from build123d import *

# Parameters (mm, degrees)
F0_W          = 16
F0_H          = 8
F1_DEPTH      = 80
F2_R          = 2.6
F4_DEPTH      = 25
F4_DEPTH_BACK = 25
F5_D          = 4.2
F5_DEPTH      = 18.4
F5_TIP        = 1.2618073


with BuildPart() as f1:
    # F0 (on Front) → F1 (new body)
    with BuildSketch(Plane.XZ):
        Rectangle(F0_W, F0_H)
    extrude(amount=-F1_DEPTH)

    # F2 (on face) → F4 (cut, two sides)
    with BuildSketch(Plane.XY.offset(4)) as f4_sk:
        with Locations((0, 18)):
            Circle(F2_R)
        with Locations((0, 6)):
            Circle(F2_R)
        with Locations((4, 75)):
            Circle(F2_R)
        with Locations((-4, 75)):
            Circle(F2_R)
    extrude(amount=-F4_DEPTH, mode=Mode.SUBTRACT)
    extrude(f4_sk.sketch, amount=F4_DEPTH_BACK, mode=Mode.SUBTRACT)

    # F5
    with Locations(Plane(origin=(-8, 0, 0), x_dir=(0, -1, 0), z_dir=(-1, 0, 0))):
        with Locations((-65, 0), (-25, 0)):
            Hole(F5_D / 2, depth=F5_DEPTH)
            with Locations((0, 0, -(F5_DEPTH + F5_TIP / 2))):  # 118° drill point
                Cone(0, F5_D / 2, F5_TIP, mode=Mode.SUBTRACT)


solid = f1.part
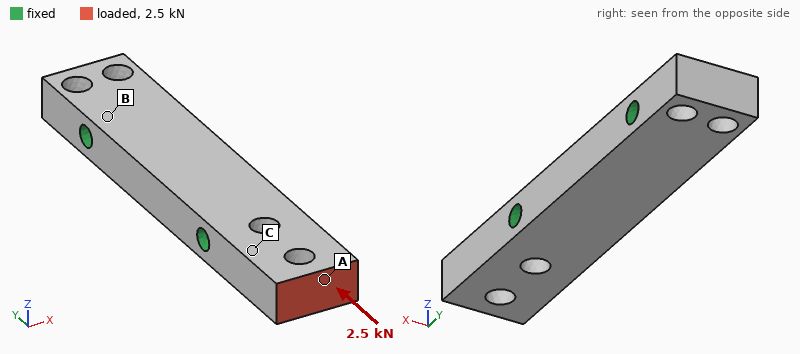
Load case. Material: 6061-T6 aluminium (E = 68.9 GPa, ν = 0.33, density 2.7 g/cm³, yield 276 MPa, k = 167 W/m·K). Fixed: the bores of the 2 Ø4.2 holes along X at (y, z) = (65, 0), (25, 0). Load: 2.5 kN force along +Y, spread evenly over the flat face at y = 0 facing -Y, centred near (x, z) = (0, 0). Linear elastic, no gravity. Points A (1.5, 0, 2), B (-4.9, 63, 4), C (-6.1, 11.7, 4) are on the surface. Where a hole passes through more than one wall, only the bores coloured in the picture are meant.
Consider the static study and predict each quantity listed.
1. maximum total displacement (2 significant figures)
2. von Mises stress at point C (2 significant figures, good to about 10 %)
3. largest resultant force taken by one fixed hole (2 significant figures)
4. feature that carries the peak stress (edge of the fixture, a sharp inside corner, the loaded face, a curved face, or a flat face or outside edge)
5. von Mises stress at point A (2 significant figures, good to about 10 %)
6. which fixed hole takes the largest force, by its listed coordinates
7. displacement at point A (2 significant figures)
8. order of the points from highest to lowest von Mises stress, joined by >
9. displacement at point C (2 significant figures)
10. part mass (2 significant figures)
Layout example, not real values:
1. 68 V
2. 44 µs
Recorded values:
1. 11 µm
2. 27 MPa
3. 2.5 kN
4. a curved face
5. 18 MPa
6. (25, 0)
7. 10 µm
8. C > A > B
9. 4.7 µm
10. 25 g
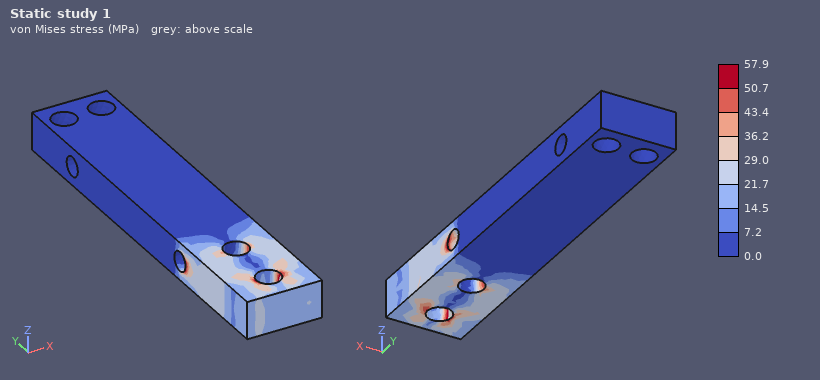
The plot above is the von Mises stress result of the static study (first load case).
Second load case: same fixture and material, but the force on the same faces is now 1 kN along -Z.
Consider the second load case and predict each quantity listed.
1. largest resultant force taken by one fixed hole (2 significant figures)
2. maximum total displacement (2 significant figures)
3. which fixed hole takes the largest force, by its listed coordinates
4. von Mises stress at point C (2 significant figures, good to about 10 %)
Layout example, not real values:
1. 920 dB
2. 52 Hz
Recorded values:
1. 1.1 kN
2. 0.16 mm
3. (25, 0)
4. 86 MPa
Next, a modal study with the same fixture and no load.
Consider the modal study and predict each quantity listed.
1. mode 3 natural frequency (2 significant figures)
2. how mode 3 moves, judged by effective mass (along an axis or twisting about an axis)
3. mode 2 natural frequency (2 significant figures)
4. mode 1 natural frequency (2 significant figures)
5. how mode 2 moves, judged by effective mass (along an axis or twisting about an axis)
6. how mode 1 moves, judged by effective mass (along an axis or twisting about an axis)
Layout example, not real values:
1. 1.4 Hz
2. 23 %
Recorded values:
1. 21 kHz
2. along Z
3. 17 kHz
4. 9200 Hz
5. along X
6. along Z
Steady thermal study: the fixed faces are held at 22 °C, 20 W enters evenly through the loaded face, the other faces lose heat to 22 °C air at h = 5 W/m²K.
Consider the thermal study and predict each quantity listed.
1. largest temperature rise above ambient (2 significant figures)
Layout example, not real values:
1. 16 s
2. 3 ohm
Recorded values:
1. 28 K
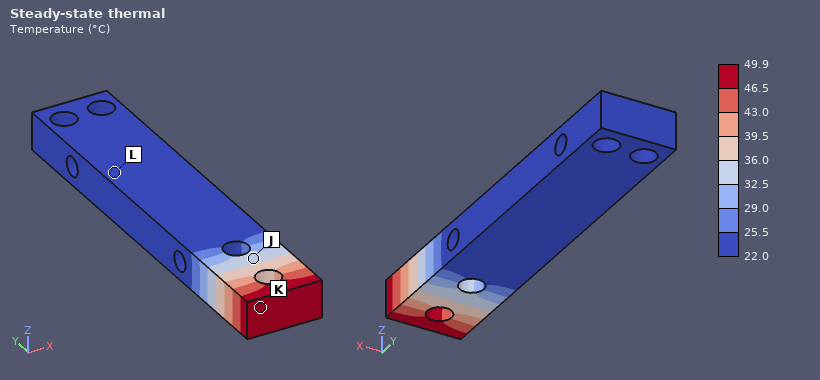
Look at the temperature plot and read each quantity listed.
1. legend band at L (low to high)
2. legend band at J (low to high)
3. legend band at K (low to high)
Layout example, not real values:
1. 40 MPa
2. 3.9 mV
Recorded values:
1. 22.0 to 25.5 °C
2. 32.5 to 36.0 °C
3. 46.5 to 49.9 °C
